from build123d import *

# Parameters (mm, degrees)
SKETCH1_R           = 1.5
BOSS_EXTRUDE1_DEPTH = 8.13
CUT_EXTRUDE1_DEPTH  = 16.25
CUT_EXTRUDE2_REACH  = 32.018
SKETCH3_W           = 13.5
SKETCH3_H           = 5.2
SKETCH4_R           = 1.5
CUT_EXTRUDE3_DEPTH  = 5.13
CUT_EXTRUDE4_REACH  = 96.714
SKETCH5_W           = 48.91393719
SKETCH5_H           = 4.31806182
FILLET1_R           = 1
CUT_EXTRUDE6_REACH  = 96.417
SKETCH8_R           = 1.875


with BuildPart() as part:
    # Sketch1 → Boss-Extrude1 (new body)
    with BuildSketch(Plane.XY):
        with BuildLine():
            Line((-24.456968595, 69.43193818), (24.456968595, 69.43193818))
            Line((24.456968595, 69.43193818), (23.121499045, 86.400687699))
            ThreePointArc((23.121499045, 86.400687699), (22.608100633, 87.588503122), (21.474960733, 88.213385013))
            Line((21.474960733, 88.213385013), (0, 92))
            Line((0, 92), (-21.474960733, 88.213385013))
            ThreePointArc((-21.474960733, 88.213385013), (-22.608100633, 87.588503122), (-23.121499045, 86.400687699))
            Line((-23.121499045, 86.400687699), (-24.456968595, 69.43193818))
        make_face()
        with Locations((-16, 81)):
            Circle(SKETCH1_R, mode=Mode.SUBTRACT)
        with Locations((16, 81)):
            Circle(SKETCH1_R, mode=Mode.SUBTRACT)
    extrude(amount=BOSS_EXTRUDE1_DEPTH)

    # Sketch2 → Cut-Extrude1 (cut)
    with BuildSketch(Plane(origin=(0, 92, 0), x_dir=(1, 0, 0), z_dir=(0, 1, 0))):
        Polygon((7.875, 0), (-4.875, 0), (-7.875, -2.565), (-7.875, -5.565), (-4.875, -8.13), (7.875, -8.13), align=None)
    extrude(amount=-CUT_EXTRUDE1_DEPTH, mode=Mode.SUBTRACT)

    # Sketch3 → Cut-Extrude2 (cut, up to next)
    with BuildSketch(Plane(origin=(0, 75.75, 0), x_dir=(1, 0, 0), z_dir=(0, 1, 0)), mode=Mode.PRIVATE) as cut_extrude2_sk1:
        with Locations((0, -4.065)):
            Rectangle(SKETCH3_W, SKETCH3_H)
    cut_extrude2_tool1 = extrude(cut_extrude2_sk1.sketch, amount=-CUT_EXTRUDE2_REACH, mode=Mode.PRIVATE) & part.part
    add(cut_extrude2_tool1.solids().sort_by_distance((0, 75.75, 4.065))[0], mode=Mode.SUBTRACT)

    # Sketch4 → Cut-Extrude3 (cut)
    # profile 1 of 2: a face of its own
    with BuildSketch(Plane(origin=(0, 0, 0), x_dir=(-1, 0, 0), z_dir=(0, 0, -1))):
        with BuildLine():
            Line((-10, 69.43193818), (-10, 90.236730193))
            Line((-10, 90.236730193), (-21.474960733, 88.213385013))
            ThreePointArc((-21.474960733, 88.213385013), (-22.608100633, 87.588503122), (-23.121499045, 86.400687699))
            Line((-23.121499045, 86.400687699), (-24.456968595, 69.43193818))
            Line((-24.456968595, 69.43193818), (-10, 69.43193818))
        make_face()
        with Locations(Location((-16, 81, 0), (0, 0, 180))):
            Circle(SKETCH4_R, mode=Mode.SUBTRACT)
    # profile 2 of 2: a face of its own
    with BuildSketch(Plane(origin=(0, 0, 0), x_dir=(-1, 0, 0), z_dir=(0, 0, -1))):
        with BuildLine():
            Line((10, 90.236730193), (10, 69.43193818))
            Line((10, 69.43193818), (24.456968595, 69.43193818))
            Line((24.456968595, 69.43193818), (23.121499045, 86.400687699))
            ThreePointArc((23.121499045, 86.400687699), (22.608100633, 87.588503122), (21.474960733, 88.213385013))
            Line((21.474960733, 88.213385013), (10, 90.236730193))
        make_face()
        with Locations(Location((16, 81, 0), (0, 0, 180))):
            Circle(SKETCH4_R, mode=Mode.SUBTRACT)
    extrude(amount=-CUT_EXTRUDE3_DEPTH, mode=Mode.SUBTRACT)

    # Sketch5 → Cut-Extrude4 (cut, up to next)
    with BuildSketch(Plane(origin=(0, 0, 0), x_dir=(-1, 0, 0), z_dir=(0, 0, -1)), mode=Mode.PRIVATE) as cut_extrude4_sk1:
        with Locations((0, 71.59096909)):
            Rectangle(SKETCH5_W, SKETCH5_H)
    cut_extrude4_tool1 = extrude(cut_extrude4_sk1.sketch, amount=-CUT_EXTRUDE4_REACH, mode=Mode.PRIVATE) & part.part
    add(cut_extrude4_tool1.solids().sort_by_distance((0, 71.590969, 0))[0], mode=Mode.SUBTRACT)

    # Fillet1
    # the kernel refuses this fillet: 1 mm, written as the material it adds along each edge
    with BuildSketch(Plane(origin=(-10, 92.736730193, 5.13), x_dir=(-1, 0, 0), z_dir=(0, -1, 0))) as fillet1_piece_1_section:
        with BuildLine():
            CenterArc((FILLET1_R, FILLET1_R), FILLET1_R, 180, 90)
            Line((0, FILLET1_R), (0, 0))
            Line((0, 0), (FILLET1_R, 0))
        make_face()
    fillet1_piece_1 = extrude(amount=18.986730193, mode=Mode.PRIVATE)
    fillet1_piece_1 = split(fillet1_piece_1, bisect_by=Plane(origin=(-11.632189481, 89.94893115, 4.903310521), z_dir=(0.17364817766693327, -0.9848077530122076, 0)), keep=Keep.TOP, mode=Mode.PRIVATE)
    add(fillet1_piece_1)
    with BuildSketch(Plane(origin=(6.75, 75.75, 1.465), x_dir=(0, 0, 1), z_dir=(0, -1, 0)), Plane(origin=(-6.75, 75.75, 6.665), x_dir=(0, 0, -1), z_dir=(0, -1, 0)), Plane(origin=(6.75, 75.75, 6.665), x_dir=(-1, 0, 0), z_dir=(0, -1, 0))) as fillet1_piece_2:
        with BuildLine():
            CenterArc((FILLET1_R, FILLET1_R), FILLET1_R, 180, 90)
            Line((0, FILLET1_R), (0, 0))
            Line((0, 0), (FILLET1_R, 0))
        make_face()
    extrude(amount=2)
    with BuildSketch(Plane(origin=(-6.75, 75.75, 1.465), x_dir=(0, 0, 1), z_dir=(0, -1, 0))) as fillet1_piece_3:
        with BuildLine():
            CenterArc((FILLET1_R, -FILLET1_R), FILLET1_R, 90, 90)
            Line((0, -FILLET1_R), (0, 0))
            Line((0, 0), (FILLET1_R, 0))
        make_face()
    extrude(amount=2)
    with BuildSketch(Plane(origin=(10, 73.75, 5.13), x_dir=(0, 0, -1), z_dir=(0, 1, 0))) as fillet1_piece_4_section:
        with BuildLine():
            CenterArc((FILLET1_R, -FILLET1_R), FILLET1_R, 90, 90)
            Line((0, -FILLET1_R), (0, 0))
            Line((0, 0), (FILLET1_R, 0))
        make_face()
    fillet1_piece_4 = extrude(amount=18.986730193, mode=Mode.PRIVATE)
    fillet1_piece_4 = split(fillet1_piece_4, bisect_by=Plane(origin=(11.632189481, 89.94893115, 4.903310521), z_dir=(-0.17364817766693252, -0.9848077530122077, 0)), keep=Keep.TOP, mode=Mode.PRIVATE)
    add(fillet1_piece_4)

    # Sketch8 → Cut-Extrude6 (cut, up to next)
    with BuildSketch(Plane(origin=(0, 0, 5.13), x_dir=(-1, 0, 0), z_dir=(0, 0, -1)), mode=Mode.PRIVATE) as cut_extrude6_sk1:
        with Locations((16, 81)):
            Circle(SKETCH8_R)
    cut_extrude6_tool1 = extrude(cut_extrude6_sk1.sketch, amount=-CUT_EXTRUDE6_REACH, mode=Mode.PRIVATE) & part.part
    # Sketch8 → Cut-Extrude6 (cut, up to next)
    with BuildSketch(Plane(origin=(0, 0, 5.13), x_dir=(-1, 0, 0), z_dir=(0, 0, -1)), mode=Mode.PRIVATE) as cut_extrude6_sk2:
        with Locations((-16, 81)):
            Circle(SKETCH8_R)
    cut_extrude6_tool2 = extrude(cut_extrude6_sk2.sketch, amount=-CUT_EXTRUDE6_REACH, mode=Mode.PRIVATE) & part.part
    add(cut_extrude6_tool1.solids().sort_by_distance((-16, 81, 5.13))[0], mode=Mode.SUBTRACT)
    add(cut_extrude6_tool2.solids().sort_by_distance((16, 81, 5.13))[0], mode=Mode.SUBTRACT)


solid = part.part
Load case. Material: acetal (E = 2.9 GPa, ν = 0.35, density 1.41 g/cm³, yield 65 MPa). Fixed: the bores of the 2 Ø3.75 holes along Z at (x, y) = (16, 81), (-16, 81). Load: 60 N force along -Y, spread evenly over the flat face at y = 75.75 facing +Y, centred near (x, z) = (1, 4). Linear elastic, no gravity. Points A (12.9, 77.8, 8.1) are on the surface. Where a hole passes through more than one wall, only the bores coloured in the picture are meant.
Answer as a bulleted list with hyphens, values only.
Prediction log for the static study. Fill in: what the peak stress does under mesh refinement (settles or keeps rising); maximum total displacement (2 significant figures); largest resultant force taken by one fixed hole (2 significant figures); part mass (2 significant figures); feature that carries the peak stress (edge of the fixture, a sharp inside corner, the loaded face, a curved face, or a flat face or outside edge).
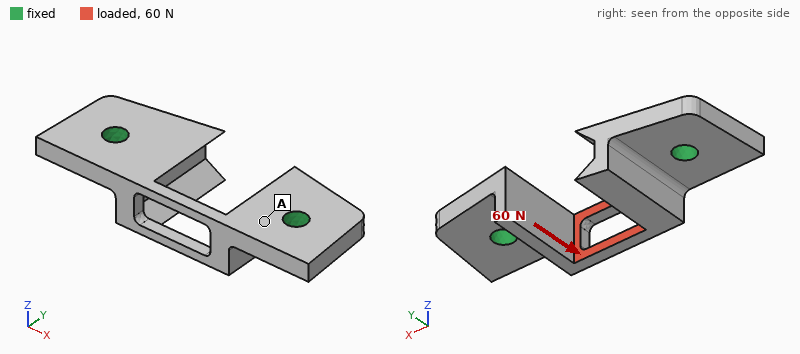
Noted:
- keeps rising
- 0.15 mm
- 36 N
- 2.8 g
- a sharp inside corner
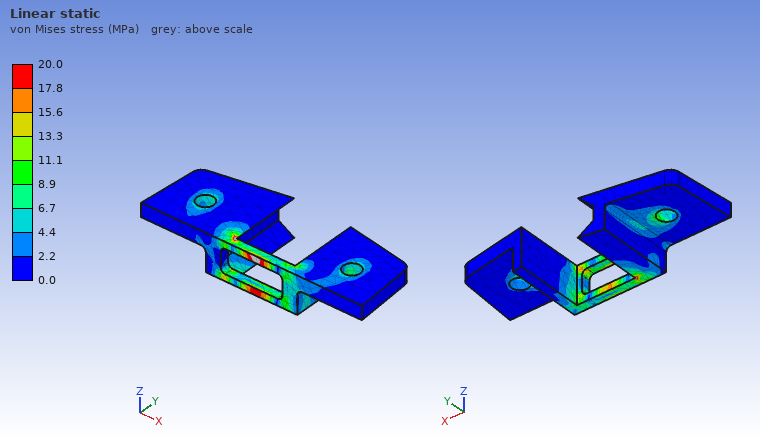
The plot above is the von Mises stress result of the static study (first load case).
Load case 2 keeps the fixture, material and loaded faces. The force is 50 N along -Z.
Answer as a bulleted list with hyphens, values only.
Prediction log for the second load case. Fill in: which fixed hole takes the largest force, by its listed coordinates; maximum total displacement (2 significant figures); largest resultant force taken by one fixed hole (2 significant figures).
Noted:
- (16, 81)
- 0.20 mm
- 29 N
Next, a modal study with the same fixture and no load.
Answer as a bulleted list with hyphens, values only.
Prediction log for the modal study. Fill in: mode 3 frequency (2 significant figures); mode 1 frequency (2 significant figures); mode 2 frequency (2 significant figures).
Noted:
- 5500 Hz
- 4400 Hz
- 5100 Hz
